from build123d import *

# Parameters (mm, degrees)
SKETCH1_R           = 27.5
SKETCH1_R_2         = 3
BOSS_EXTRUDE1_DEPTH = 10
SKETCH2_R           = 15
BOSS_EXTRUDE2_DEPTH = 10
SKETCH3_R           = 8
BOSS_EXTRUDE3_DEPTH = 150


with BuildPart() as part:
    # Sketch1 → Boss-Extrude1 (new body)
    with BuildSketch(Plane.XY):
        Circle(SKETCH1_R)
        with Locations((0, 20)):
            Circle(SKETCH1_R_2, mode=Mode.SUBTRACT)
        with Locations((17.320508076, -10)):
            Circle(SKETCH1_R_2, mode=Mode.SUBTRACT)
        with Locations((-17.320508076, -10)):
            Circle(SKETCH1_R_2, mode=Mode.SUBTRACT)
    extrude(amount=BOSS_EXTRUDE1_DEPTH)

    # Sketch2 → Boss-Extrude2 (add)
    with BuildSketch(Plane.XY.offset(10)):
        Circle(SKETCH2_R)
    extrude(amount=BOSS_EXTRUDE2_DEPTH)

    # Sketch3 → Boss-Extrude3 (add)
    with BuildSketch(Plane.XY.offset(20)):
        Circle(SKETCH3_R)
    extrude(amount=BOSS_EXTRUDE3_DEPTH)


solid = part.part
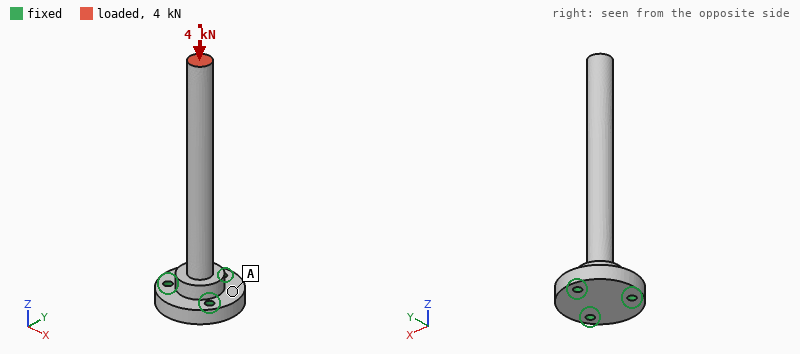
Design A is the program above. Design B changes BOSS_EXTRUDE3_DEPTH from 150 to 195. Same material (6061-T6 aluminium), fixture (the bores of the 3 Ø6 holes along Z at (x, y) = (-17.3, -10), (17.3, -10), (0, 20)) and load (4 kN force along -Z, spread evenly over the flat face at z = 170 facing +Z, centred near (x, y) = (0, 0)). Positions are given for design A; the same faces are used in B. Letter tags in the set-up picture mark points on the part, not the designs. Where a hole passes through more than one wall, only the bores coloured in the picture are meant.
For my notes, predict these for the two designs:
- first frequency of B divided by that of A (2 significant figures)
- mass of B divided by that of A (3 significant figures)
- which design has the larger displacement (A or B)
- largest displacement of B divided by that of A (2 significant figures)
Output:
0.60
1.15
B
1.3
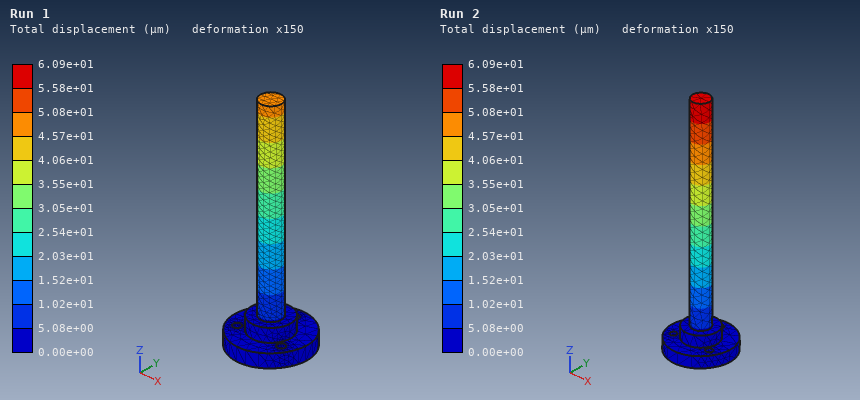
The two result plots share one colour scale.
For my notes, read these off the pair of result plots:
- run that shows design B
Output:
Run 2
